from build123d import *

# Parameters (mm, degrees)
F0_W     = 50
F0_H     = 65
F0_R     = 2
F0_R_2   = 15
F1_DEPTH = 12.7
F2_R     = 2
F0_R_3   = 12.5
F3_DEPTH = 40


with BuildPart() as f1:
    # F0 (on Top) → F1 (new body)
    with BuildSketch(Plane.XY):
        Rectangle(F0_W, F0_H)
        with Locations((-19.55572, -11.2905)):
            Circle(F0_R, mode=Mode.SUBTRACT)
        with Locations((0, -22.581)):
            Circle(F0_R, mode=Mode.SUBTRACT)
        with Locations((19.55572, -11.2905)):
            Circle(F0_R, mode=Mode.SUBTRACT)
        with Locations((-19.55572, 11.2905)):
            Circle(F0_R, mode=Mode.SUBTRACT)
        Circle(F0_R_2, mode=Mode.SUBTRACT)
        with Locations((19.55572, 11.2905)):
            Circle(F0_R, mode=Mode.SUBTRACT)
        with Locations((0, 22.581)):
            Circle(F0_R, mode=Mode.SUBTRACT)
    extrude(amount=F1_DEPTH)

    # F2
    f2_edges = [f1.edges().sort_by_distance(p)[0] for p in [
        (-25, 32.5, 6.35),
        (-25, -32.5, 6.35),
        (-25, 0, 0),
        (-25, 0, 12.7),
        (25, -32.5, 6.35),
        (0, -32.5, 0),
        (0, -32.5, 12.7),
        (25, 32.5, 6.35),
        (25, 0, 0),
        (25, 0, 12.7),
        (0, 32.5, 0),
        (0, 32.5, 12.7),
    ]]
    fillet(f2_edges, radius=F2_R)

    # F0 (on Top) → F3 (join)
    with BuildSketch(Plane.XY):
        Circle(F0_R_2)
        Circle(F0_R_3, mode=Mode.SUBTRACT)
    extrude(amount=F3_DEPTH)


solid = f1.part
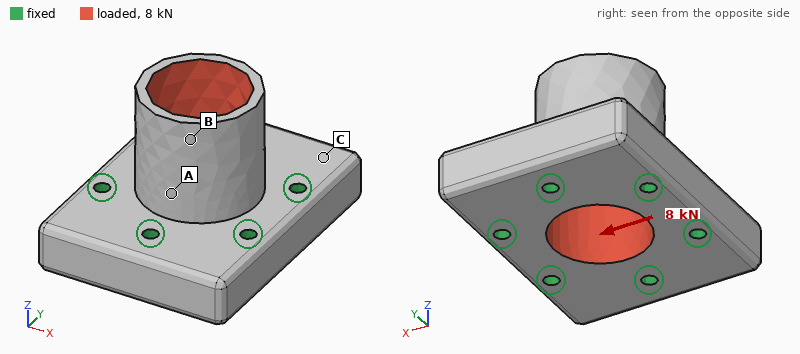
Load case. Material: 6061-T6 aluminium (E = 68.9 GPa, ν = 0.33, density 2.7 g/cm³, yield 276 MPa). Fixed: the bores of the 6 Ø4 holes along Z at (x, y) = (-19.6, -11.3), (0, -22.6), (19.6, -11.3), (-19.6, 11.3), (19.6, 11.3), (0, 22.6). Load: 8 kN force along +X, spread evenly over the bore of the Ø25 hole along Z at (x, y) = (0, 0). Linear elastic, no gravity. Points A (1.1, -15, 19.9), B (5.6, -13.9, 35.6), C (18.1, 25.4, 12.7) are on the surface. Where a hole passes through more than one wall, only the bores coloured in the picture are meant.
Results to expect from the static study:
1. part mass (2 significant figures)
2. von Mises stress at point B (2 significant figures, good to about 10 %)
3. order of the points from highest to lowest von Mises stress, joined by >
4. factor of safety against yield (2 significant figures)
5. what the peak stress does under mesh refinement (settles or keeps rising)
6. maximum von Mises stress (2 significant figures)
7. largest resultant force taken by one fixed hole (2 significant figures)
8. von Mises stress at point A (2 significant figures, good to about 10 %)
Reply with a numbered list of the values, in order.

1. 110 g
2. 14 MPa
3. A > B > C
4. 3.5
5. settles
6. 79 MPa
7. 2.2 kN
8. 52 MPa
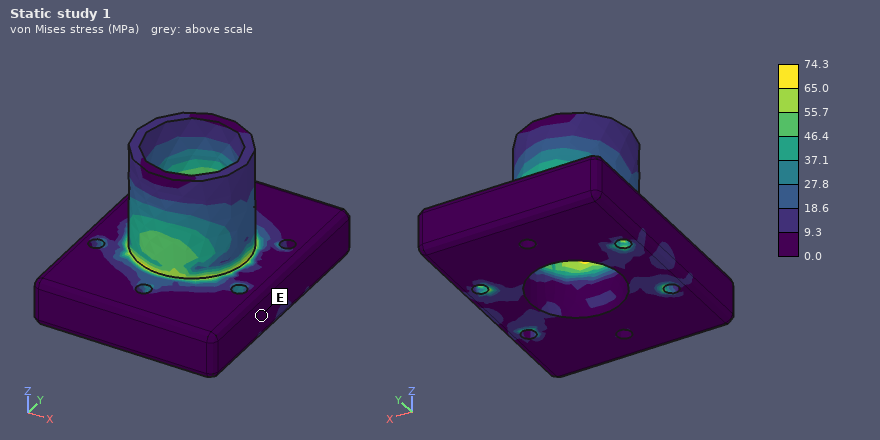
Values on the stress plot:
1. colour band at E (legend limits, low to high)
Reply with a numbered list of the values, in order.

1. 0.0 to 9.3 MPa
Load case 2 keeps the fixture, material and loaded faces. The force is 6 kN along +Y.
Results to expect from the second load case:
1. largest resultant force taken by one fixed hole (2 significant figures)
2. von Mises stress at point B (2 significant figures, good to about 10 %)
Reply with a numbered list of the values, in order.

1. 1.9 kN
2. 10 MPa
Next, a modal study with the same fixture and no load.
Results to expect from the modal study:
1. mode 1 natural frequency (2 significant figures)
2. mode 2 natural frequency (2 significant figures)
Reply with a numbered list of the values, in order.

1. 13 kHz
2. 13 kHz
